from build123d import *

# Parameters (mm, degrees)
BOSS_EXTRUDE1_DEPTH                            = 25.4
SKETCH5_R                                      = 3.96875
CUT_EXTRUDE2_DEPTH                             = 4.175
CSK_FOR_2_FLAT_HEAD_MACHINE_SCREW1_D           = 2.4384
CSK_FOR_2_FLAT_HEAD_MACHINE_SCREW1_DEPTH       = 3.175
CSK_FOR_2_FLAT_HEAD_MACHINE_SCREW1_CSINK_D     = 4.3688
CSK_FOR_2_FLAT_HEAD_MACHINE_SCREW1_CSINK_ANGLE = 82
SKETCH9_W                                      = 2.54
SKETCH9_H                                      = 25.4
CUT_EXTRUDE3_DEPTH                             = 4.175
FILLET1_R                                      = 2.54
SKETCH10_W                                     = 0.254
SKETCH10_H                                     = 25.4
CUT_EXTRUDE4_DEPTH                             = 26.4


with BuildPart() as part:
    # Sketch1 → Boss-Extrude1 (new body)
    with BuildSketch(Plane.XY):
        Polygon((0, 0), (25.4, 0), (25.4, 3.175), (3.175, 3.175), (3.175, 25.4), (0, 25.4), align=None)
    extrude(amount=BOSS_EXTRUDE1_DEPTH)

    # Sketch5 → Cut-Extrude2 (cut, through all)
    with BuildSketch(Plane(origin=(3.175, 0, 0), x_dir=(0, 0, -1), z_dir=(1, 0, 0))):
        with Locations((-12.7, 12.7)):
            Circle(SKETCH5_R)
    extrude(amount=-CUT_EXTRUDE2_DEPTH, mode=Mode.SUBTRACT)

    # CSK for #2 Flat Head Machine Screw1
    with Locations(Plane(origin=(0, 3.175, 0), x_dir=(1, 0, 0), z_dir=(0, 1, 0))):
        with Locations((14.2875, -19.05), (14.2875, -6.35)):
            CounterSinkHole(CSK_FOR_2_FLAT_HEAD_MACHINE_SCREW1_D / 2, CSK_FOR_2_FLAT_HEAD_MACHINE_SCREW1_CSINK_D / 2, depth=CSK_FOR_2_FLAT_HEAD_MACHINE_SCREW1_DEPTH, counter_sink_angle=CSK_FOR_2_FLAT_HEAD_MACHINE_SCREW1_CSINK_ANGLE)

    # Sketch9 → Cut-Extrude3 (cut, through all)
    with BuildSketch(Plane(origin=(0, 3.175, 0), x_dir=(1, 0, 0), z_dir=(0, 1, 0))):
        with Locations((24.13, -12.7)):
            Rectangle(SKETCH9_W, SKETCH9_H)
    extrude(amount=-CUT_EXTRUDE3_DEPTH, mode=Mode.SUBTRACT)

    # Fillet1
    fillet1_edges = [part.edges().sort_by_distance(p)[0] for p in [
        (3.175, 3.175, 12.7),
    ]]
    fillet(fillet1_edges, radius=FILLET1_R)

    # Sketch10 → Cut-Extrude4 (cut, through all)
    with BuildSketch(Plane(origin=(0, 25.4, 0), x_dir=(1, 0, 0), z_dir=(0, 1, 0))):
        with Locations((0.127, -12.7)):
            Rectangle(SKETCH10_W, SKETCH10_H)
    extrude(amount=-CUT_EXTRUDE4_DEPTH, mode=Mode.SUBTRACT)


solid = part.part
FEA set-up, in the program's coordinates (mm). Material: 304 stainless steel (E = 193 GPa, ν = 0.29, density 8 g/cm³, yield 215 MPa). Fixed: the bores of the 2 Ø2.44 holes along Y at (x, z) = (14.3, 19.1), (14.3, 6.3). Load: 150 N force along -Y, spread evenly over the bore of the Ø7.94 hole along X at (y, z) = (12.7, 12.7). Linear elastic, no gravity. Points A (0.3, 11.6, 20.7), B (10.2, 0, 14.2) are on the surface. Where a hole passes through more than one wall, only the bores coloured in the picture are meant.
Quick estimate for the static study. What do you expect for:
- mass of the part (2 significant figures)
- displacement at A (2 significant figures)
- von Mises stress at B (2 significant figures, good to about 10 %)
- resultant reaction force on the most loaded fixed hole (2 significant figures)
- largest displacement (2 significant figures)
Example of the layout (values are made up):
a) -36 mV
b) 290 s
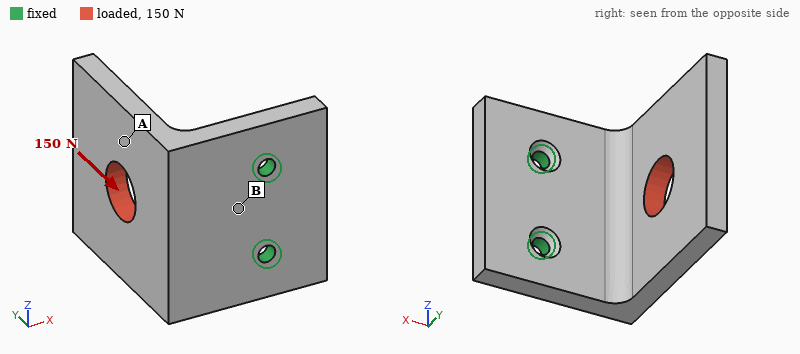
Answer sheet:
a) 27 g
b) 18 µm
c) 26 MPa
d) 75 N
e) 32 µm
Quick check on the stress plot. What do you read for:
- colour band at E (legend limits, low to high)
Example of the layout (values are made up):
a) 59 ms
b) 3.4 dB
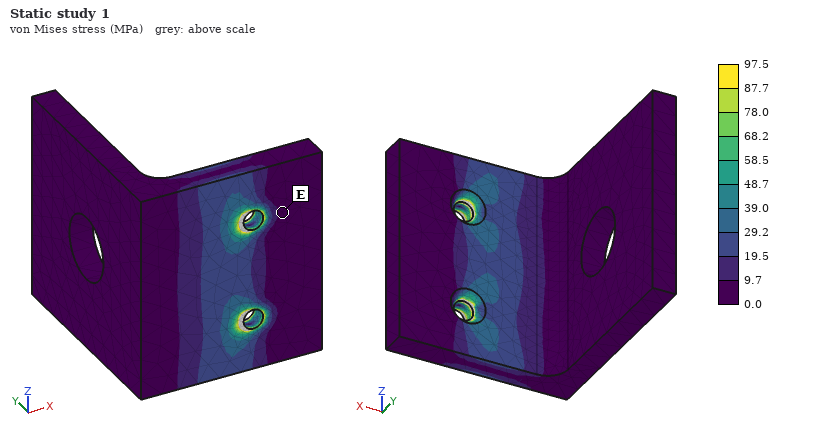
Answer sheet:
a) 0.0 to 9.7 MPa
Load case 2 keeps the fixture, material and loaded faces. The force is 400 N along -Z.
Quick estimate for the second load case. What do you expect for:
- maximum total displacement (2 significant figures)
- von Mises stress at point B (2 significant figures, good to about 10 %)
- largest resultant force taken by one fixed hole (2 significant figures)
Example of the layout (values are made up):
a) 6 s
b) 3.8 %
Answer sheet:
a) 41 µm
b) 35 MPa
c) 510 N
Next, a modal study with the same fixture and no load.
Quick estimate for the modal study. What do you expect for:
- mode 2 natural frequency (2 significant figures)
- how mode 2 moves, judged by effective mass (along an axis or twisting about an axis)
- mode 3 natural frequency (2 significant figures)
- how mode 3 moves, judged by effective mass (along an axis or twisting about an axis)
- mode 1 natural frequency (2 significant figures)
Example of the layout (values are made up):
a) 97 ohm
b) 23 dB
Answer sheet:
a) 4600 Hz
b) along Z
c) 7200 Hz
d) along Y
e) 2400 Hz
